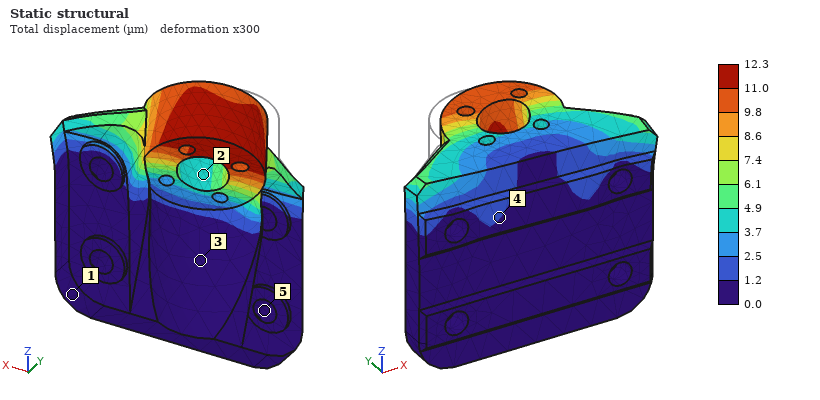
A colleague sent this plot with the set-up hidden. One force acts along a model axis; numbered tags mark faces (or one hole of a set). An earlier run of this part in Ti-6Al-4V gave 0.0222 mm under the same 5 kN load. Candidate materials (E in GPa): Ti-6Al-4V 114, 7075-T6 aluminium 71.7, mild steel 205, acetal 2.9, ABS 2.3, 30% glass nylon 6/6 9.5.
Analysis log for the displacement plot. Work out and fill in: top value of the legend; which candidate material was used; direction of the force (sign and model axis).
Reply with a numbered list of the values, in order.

1. 12.3 µm
2. mild steel
3. +X
